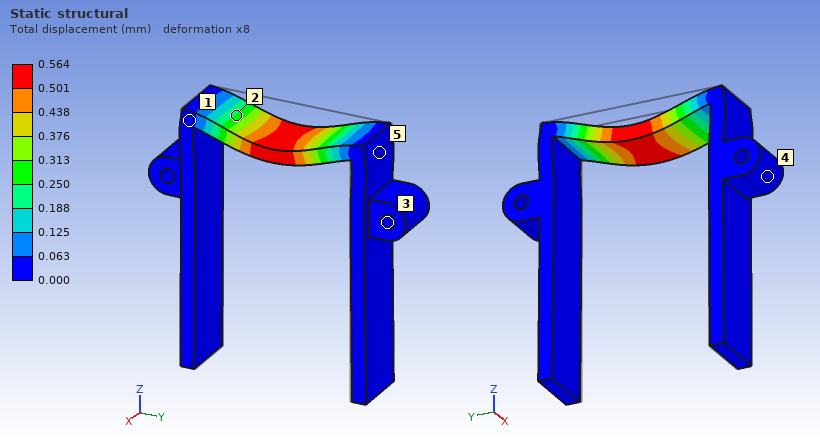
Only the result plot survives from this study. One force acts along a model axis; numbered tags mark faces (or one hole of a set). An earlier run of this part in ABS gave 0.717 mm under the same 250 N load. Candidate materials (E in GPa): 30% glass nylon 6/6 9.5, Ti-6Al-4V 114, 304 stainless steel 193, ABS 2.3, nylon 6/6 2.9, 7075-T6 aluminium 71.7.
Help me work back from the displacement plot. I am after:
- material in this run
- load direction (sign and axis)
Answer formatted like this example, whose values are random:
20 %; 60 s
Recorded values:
nylon 6/6; -Z
